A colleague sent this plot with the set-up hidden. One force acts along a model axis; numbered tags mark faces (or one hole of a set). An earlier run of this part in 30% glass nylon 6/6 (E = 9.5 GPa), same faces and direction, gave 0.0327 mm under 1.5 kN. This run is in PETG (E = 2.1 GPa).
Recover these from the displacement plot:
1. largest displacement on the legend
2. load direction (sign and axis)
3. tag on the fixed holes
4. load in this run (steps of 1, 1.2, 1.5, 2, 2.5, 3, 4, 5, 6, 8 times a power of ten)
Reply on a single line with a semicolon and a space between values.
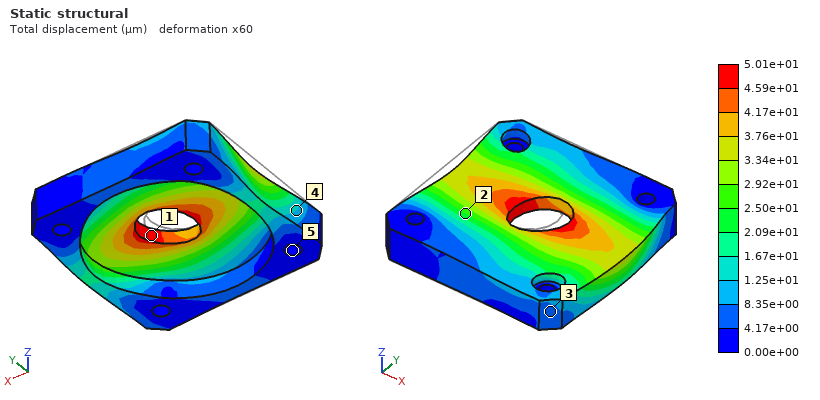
5.01e+01 µm; +X; 5; 500 N
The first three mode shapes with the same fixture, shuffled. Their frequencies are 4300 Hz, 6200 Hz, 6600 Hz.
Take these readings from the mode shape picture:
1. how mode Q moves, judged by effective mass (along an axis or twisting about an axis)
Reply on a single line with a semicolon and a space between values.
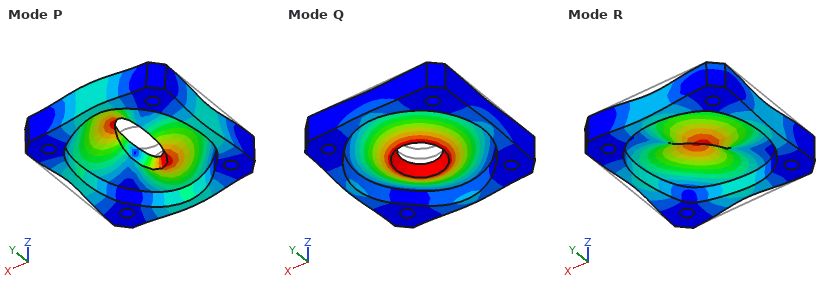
along Z
